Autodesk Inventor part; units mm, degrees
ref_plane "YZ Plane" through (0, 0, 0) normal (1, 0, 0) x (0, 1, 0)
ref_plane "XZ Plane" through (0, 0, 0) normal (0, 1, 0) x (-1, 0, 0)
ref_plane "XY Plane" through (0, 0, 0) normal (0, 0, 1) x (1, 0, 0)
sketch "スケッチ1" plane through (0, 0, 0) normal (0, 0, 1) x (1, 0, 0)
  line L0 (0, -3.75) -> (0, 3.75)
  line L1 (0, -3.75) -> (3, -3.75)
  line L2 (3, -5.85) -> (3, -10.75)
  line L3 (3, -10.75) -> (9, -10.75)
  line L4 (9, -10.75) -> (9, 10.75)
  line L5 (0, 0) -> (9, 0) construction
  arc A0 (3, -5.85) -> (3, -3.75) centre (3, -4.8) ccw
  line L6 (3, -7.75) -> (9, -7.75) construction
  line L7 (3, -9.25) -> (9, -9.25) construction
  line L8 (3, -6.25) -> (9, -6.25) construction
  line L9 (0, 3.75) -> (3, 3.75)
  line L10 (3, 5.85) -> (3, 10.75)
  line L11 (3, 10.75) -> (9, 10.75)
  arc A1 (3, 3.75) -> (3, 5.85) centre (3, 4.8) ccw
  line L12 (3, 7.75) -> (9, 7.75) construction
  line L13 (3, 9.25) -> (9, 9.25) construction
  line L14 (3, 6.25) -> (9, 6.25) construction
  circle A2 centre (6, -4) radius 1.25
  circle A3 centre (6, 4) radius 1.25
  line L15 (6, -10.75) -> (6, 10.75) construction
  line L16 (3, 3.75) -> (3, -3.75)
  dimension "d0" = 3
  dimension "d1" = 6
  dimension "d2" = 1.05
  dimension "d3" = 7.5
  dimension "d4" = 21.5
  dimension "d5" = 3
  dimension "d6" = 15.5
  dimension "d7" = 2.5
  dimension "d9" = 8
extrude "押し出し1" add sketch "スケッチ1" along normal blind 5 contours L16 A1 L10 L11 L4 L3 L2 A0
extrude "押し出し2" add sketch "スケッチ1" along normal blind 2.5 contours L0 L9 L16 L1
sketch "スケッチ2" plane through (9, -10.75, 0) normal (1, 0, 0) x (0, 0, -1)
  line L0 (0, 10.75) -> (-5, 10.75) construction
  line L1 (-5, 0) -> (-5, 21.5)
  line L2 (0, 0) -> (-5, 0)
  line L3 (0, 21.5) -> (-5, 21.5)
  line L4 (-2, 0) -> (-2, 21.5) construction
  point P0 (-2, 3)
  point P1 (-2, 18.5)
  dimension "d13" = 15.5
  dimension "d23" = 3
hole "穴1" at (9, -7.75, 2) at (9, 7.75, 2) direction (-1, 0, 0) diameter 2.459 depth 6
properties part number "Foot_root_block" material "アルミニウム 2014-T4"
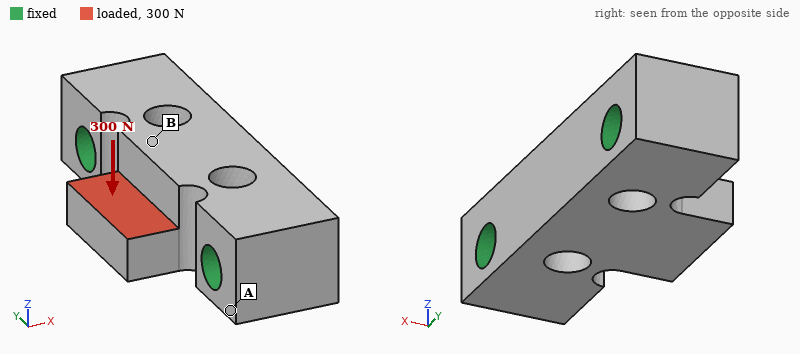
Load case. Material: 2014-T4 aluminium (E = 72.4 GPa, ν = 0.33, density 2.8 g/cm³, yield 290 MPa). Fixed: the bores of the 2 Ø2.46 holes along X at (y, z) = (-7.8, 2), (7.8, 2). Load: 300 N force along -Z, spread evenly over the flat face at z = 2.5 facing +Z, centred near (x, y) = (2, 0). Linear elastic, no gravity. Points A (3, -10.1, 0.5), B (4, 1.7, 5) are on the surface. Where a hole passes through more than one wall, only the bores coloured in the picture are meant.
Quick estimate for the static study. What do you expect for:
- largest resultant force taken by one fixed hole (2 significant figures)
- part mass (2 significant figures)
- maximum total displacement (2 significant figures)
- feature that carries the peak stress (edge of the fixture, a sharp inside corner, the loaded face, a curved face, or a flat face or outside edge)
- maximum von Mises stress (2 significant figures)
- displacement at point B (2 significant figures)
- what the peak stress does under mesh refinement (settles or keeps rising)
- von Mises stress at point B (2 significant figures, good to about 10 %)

150 N
1.6 g
24 µm
a curved face
190 MPa
9.3 µm
settles
34 MPa
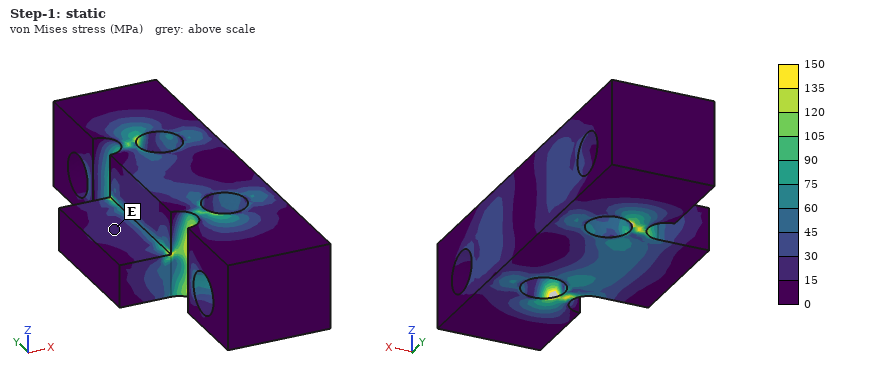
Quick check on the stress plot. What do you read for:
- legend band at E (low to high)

15 to 30 MPa
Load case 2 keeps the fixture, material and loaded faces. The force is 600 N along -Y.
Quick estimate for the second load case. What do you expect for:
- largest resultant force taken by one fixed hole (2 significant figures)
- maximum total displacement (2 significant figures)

360 N
15 µm
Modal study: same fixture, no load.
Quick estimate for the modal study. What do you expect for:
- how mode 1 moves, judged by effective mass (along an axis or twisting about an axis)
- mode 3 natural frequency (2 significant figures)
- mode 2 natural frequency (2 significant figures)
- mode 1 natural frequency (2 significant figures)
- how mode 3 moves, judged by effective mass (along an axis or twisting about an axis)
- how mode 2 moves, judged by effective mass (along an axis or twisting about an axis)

along Z
73 kHz
59 kHz
42 kHz
along Z
along X
